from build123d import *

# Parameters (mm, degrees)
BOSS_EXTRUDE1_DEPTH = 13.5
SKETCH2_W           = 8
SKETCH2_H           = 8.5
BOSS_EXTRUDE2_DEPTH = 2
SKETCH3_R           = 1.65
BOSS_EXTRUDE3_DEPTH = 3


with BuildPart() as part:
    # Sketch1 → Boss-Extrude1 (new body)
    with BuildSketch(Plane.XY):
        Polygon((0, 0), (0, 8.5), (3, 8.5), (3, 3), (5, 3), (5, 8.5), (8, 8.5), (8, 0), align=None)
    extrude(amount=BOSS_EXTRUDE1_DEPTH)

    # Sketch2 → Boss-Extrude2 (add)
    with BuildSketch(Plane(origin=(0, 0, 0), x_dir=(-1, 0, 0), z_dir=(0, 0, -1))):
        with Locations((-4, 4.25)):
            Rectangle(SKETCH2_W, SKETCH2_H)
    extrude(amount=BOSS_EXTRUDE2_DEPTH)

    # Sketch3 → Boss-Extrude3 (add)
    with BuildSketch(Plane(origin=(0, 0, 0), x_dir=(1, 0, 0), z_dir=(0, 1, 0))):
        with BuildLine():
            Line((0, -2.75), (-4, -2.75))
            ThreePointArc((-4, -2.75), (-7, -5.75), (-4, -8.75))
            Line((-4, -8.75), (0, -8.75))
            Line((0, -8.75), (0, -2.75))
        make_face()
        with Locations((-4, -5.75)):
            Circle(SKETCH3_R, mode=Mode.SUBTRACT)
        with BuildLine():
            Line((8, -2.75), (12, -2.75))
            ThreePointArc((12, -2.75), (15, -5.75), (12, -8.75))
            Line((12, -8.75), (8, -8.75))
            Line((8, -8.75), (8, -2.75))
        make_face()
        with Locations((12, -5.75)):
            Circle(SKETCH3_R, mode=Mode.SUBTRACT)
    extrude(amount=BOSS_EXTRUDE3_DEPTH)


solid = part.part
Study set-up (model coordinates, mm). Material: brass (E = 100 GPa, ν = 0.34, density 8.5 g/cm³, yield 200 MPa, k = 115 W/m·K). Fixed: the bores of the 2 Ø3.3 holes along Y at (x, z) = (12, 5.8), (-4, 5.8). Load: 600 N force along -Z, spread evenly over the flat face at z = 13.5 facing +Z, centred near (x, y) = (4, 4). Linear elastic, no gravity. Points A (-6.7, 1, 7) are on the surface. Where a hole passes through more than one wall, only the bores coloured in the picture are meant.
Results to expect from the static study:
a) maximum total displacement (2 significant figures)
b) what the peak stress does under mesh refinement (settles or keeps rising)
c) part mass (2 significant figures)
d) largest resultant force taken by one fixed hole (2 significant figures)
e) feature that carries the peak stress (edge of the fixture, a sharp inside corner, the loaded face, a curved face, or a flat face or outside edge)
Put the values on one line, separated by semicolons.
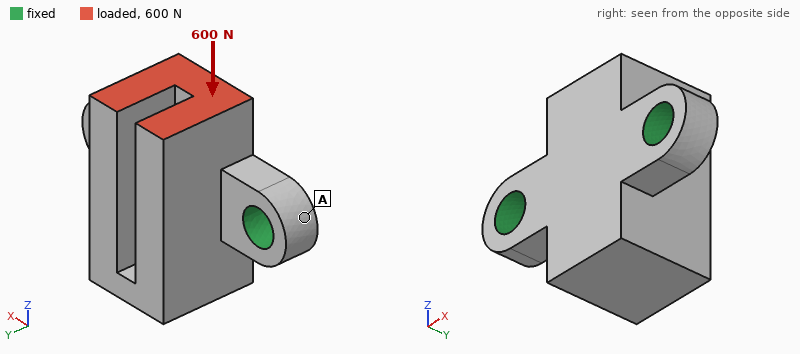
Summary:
20 µm; keeps rising; 9.2 g; 300 N; edge of the fixture
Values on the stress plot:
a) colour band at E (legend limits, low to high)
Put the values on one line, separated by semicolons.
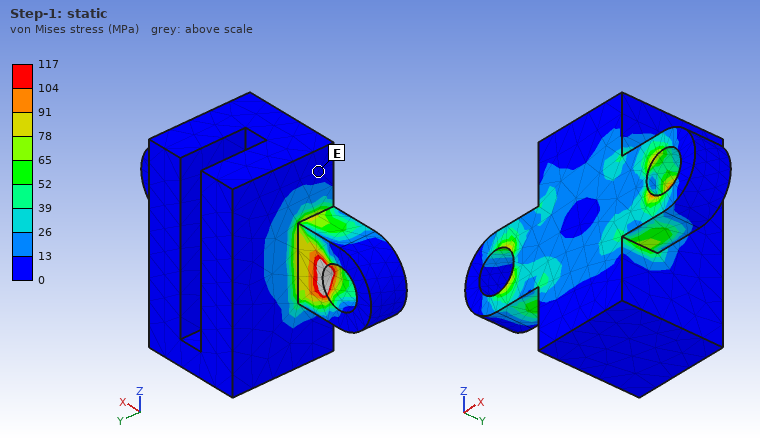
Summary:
0 to 13 MPa
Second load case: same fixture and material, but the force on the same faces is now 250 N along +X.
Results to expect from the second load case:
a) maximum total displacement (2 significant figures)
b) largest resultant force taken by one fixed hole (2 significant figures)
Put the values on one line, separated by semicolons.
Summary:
7.8 µm; 200 N
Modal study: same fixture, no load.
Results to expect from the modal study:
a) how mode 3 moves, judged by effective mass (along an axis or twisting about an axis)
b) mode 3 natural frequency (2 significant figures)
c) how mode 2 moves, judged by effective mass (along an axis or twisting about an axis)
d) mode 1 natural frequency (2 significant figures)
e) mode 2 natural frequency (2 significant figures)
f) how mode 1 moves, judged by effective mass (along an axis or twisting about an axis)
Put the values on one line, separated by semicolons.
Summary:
along X; 25 kHz; along Y; 9400 Hz; 21 kHz; along Z
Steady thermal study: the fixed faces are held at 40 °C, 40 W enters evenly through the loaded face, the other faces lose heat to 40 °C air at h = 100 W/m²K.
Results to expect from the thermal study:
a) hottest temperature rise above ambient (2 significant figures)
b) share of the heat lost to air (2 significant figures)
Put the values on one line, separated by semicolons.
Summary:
79 K; 8.0 %
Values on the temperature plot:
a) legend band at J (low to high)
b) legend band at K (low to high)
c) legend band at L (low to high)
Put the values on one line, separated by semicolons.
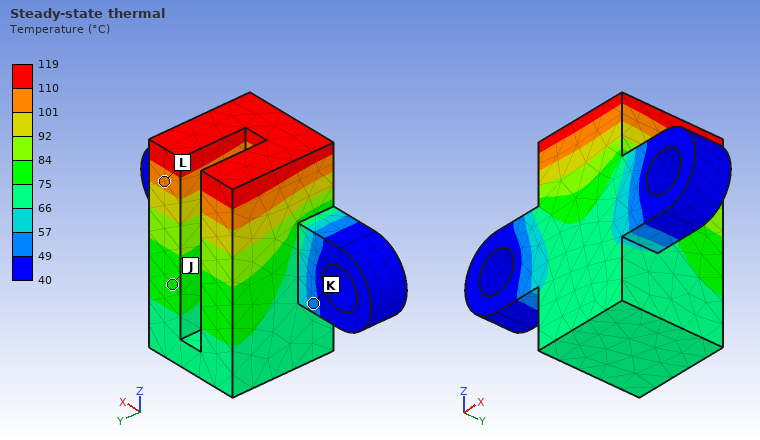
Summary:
75 to 84 °C; 49 to 57 °C; 101 to 110 °C
